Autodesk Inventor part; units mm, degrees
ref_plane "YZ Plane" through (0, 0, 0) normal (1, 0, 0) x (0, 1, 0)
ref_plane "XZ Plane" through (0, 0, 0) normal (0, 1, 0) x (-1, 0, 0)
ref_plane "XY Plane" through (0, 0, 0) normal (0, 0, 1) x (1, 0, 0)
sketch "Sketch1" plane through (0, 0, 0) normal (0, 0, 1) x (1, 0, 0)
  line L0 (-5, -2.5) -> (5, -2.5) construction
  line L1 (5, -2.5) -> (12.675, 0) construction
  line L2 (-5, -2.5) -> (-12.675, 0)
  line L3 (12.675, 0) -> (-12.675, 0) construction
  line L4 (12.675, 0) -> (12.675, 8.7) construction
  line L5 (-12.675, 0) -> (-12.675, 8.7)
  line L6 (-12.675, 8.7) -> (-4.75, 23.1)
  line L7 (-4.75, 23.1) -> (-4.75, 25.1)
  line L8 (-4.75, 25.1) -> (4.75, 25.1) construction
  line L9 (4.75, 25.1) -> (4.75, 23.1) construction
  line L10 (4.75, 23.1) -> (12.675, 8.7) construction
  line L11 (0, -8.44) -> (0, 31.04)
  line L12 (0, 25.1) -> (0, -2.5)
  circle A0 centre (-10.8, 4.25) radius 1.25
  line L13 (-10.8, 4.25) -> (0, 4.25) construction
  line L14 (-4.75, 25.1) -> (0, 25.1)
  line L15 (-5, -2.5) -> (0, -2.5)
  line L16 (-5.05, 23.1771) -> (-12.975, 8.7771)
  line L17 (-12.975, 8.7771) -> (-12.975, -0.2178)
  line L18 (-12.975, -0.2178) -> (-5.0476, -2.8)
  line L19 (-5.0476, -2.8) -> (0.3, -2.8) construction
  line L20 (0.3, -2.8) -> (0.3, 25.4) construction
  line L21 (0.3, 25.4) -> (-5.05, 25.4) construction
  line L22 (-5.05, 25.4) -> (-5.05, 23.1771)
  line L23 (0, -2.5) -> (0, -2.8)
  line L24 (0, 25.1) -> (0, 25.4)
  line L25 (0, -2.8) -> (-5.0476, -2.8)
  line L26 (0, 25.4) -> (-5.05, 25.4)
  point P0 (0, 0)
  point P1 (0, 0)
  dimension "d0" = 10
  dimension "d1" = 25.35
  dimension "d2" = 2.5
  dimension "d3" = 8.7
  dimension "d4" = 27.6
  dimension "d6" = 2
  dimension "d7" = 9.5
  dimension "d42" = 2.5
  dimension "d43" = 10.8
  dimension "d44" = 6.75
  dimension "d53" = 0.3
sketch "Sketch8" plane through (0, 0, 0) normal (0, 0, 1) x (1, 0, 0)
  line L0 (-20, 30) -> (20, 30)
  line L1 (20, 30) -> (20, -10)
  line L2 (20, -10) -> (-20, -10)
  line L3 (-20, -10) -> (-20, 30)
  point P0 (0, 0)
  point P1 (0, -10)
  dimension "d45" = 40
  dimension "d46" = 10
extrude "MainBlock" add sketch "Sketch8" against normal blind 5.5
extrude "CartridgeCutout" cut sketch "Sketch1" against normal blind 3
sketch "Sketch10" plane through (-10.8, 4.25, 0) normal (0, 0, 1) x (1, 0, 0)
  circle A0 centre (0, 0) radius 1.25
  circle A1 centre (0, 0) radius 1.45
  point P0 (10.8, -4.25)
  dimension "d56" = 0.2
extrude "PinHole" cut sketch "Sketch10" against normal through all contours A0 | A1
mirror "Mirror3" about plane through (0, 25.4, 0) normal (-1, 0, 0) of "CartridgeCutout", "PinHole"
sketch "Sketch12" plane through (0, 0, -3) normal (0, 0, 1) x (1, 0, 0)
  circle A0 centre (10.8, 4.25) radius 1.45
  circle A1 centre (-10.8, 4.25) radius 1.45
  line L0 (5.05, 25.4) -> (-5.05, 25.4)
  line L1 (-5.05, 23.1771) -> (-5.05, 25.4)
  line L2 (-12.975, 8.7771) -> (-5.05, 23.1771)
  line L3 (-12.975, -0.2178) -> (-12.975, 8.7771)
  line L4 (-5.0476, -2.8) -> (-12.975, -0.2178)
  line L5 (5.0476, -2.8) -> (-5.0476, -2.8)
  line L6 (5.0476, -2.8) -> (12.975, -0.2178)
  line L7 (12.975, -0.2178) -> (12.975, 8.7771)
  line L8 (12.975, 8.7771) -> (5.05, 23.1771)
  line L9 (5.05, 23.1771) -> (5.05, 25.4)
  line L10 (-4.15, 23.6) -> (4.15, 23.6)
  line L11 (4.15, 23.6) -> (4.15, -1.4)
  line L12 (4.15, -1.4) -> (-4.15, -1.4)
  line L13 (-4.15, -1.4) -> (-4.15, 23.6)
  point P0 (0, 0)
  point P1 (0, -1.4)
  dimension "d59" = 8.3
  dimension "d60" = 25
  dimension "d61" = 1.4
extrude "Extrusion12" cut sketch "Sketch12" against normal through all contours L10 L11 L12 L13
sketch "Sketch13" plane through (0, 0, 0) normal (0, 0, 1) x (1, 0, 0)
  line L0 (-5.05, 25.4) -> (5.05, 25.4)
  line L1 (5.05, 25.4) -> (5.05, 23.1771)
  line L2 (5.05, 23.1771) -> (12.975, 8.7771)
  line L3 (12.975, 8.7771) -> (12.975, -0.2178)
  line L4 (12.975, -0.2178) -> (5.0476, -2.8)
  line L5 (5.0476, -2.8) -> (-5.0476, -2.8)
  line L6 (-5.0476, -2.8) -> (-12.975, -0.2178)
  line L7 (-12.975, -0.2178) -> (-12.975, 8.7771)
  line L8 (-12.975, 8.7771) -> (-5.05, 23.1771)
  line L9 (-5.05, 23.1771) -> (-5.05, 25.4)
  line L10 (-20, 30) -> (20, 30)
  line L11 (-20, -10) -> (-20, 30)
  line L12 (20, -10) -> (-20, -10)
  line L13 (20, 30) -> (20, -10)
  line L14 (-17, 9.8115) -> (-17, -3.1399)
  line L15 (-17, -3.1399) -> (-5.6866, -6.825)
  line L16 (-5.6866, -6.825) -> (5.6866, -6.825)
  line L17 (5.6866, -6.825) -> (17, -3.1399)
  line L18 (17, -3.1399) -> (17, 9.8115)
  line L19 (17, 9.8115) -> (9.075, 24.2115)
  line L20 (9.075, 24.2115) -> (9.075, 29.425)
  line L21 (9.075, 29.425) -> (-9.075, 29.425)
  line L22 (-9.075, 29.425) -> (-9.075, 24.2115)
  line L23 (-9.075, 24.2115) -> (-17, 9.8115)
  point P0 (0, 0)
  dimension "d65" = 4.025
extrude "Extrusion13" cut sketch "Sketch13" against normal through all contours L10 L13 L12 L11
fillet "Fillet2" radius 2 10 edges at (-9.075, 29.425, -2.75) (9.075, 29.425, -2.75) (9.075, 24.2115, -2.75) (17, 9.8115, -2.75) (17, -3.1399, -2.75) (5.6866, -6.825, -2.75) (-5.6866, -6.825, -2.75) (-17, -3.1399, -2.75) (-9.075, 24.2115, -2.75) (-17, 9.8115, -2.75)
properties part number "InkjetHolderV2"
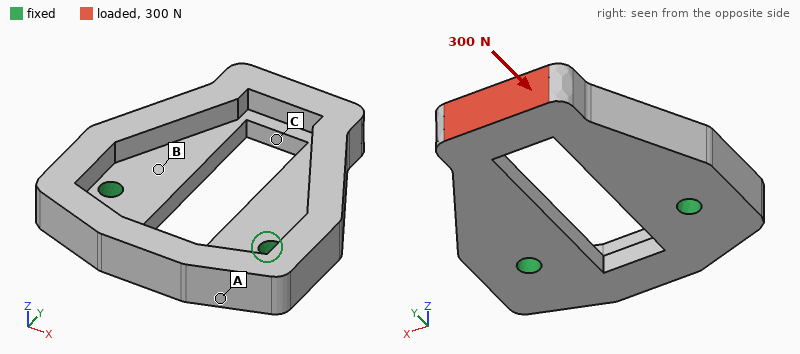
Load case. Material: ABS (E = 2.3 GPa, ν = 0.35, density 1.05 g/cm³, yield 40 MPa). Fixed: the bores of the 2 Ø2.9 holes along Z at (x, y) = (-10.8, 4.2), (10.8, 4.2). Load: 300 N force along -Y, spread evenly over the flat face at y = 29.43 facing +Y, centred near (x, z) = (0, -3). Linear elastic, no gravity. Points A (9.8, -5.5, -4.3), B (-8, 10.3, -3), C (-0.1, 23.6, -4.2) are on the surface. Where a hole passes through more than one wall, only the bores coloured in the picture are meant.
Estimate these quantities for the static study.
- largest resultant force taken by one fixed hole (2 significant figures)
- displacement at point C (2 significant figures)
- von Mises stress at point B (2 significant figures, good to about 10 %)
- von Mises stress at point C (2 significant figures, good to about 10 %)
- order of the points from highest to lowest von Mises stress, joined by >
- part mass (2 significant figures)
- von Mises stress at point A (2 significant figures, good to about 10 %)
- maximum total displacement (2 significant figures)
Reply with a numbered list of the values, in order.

1. 160 N
2. 0.30 mm
3. 8.2 MPa
4. 12 MPa
5. C > B > A
6. 3.4 g
7. 2.6 MPa
8. 0.49 mm
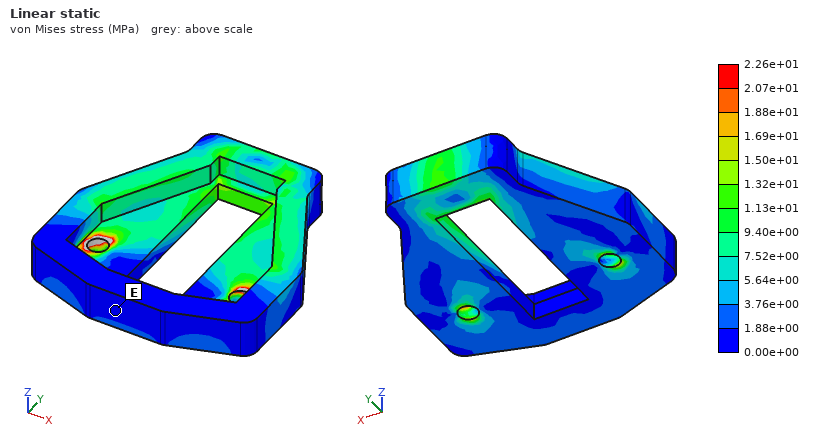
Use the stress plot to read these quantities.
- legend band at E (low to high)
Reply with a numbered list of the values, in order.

1. 0.00e+00 to 1.88e+00 MPa
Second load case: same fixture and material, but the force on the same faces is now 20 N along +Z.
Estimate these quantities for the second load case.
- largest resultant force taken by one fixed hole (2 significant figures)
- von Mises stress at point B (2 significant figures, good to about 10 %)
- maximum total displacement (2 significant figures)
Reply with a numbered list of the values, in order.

1. 17 N
2. 3.1 MPa
3. 0.52 mm
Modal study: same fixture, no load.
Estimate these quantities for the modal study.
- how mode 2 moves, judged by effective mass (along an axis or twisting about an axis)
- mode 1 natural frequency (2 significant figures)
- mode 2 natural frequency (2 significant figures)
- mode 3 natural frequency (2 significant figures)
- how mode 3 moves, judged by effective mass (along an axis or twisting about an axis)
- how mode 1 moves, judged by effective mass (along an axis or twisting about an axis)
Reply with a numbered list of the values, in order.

1. along X
2. 1300 Hz
3. 3300 Hz
4. 3800 Hz
5. along X
6. along Z
